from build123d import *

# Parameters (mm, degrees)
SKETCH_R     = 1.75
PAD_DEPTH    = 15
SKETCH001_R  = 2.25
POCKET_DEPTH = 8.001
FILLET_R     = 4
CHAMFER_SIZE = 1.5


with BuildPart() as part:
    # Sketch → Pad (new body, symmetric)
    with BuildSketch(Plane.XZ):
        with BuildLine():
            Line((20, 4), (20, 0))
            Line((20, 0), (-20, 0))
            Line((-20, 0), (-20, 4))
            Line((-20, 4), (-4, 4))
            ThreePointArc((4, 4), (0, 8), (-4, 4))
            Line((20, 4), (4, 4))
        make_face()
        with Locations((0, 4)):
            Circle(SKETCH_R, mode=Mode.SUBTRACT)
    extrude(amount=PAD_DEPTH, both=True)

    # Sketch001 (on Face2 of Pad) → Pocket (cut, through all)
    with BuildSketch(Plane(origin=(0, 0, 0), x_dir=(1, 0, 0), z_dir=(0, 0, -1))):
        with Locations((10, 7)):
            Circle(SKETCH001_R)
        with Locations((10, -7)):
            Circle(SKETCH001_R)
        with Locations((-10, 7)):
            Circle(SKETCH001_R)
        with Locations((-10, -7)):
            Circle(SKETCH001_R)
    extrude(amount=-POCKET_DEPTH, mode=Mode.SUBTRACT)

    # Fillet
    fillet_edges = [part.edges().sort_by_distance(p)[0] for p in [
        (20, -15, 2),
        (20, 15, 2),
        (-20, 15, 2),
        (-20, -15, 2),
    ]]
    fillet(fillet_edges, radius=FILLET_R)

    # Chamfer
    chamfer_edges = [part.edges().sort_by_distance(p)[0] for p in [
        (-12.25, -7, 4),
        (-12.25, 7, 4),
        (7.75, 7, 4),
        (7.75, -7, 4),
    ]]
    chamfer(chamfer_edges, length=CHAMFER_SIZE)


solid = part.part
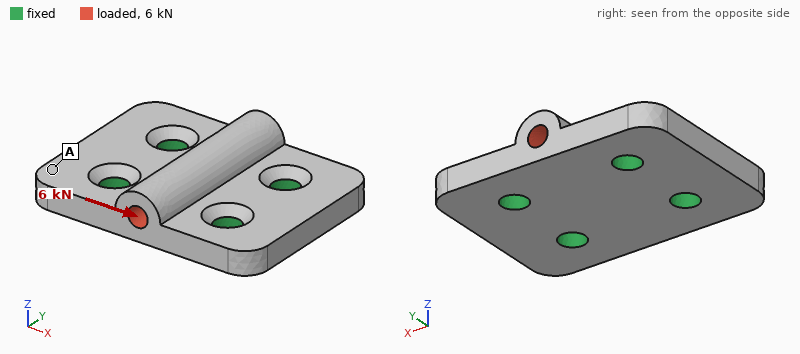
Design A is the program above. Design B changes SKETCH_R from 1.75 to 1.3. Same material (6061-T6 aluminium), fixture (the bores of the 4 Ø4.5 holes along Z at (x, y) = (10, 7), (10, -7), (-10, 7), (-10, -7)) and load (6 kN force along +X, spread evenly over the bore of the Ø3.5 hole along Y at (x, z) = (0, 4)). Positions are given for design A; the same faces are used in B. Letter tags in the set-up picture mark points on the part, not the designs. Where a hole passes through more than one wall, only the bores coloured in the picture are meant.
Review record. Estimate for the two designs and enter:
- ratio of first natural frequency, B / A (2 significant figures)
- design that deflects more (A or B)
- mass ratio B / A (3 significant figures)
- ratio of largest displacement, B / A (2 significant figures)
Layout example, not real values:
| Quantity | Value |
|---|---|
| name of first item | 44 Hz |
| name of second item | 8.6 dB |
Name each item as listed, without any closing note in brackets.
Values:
| Quantity | Value |
|---|---|
| ratio of first natural frequency, B / A | 1.0 |
| design that deflects more | A |
| mass ratio B / A | 1.03 |
| ratio of largest displacement, B / A | 0.87 |
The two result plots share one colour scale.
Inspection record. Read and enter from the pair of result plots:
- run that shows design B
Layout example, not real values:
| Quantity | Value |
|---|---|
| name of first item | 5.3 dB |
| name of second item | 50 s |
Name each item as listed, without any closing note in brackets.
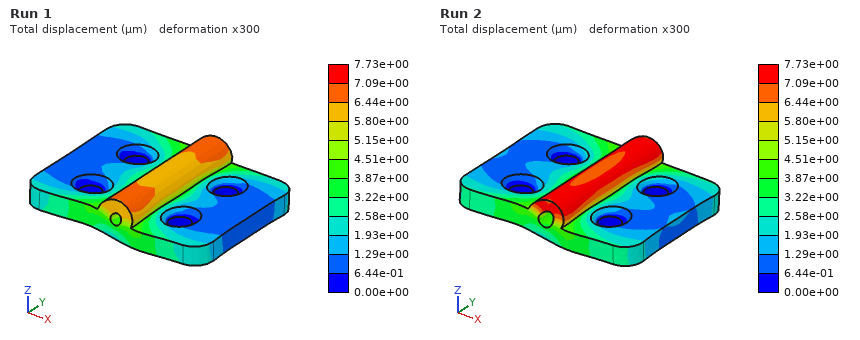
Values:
| Quantity | Value |
|---|---|
| run that shows design B | Run 1 |
